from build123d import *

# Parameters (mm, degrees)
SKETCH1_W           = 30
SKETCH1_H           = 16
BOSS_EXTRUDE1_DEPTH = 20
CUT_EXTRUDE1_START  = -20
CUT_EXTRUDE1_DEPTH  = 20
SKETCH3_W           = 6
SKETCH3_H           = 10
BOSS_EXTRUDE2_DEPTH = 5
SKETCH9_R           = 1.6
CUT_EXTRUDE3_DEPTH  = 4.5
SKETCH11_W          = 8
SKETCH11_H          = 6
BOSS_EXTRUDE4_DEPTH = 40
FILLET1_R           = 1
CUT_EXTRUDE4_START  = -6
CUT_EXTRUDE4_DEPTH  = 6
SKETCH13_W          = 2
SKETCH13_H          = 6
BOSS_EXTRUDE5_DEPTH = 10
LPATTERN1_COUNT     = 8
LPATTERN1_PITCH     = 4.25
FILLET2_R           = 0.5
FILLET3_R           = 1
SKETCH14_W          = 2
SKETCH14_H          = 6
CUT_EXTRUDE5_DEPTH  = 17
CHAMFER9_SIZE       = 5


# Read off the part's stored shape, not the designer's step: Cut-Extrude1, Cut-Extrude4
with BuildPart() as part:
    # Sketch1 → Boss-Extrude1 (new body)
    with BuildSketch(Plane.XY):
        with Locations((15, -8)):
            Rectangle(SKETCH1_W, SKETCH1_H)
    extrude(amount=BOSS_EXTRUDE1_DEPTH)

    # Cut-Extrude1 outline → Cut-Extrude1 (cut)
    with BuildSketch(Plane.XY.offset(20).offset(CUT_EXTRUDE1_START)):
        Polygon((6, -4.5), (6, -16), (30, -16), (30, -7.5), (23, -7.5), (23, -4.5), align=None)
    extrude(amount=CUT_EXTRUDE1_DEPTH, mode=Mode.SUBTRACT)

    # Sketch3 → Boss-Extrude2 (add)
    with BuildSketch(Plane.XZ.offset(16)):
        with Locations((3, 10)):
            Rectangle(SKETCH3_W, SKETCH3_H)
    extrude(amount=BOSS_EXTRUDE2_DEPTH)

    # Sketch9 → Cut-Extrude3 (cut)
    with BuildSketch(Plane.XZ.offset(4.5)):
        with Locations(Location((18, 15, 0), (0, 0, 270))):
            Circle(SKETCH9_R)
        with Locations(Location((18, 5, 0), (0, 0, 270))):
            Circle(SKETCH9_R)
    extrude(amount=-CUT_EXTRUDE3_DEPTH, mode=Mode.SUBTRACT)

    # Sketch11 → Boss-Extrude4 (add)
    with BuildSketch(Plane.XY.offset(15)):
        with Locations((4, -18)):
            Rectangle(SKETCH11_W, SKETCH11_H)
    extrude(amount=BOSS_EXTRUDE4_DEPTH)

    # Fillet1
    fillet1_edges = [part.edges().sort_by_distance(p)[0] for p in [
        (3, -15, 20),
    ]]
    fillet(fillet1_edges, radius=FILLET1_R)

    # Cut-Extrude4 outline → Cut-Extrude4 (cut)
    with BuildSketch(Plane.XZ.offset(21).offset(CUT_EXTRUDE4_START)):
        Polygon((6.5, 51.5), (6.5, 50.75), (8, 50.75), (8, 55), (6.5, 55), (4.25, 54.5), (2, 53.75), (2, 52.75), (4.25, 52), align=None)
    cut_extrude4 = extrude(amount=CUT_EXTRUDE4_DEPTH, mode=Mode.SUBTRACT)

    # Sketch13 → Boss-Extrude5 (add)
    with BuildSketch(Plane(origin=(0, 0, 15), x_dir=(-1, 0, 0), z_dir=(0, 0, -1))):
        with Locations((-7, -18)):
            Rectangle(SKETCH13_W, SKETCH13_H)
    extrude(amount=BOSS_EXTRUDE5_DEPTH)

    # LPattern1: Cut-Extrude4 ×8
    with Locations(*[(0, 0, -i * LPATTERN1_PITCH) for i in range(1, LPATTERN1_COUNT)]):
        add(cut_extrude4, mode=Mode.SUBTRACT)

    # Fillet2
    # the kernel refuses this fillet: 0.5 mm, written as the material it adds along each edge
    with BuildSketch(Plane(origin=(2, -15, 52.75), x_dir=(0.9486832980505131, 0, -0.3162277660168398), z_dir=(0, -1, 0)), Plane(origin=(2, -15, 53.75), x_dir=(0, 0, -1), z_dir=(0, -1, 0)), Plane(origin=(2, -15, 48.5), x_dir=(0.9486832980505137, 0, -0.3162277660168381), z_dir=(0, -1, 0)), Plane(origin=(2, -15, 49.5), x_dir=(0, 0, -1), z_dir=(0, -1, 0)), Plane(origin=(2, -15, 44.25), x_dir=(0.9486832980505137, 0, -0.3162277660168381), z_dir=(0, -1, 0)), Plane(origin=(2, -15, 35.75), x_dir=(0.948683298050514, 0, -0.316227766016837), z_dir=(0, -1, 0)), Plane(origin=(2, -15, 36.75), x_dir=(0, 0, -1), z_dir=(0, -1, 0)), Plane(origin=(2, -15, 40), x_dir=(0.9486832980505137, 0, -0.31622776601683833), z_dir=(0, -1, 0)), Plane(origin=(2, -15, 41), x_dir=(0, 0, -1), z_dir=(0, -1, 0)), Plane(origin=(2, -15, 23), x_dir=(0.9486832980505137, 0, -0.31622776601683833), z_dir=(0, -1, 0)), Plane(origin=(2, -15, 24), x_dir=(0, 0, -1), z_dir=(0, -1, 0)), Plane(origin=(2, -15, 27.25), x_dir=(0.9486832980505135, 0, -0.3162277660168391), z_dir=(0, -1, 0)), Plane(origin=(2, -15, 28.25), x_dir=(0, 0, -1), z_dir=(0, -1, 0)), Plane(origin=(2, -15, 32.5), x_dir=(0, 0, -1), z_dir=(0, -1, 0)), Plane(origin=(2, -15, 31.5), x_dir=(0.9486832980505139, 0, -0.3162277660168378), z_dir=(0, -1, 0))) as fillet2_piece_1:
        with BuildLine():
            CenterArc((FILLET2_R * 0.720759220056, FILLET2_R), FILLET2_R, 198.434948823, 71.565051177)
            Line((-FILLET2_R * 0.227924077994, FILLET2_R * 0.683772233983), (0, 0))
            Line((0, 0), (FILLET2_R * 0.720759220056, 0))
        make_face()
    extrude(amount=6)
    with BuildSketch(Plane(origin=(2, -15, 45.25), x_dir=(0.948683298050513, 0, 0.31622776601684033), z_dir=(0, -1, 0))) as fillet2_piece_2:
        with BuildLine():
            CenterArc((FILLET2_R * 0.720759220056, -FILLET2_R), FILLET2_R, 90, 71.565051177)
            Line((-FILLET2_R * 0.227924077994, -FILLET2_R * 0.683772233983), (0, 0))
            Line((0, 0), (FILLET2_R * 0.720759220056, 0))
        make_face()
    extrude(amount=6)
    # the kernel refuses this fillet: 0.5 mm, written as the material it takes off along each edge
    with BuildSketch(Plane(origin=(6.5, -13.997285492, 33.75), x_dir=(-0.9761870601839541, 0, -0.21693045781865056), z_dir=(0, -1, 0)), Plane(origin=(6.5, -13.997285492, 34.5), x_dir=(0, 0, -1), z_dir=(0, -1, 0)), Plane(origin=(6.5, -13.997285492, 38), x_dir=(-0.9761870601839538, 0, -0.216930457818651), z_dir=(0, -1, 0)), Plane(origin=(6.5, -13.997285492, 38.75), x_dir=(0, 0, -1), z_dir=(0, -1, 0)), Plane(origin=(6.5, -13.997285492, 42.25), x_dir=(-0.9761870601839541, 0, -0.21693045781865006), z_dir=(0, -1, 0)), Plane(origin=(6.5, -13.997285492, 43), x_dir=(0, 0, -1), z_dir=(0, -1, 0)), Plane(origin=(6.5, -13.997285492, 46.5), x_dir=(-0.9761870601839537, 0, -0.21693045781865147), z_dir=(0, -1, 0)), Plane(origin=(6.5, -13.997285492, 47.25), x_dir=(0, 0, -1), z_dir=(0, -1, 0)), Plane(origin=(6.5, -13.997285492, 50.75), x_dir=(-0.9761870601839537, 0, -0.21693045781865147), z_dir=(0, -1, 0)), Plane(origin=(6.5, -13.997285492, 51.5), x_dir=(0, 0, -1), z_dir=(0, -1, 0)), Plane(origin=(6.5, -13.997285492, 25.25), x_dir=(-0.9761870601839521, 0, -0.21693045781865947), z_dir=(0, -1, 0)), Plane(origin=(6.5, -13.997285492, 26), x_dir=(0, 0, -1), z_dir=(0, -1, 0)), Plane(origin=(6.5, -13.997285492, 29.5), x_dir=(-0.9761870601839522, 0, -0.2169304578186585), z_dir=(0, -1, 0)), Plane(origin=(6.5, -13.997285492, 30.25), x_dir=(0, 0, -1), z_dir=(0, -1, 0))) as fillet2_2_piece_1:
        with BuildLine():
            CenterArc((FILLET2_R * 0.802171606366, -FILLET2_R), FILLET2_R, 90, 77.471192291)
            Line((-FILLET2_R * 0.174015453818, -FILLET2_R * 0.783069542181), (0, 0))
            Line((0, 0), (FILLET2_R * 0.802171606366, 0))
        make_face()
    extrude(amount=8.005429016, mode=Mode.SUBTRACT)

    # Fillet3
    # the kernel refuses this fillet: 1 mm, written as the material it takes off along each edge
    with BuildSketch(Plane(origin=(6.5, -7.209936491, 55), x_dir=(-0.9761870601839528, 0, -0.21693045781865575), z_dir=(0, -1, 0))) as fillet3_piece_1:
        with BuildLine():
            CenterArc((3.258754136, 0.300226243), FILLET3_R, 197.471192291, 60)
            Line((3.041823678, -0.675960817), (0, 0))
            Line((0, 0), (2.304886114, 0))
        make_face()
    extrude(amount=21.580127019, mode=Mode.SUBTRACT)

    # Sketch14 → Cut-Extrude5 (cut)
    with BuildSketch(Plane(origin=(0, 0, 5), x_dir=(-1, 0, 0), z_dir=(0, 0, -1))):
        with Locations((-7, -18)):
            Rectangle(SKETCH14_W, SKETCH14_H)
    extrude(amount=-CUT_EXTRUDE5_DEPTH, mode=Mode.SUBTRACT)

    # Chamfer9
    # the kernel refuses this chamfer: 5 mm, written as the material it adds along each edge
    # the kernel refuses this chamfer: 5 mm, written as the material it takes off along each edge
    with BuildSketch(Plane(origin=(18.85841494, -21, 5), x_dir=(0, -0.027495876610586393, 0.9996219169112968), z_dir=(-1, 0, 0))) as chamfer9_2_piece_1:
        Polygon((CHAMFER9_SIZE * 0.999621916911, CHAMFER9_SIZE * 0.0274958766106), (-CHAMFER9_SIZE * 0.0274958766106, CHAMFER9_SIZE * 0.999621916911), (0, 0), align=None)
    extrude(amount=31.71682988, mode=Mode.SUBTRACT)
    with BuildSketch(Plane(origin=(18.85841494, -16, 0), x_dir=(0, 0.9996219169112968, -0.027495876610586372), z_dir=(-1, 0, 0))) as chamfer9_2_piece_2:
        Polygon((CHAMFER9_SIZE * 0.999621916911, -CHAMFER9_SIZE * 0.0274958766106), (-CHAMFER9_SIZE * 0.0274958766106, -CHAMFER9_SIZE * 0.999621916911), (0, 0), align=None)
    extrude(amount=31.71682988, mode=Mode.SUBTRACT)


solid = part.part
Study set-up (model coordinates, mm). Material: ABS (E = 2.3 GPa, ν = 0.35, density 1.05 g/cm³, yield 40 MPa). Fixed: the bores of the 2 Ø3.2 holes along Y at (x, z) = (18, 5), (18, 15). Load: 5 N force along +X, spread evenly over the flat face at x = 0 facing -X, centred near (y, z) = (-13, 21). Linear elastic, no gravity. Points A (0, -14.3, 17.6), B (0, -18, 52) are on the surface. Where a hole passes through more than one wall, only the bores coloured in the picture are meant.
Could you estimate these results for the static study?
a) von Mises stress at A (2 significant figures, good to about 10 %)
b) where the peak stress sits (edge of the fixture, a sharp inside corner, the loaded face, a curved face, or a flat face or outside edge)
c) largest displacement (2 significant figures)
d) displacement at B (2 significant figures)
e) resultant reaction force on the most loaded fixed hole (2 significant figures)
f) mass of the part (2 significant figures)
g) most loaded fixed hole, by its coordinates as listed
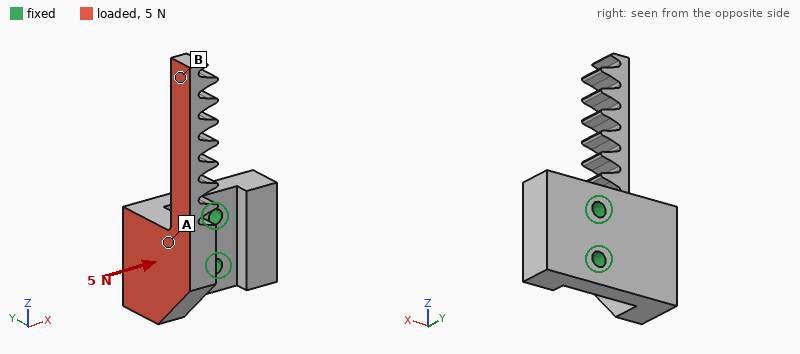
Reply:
0.85 MPa
a curved face
0.68 mm
0.60 mm
7.0 N
5.8 g
(18, 15)
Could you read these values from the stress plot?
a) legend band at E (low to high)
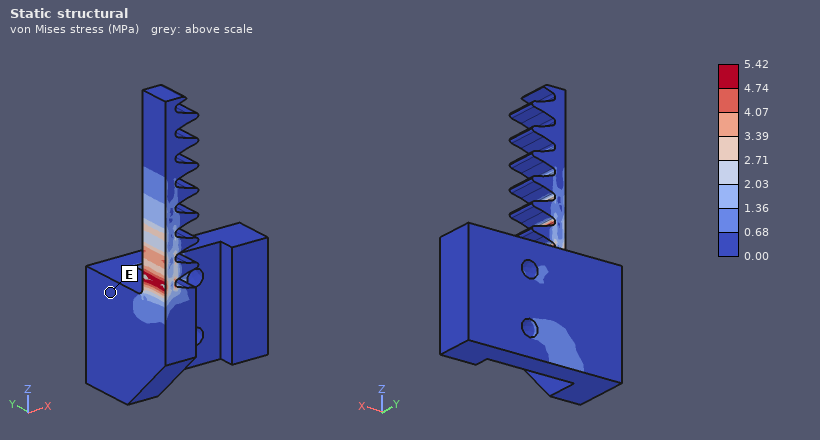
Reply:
0.00 to 0.68 MPa
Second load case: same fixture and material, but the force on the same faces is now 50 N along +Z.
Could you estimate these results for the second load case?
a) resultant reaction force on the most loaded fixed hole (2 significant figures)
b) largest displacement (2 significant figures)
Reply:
85 N
0.75 mm
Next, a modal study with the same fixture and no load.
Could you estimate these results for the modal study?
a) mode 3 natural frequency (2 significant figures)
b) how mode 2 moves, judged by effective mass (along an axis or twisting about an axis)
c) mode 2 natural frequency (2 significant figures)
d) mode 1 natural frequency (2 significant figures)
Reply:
1200 Hz
along Y
680 Hz
360 Hz
